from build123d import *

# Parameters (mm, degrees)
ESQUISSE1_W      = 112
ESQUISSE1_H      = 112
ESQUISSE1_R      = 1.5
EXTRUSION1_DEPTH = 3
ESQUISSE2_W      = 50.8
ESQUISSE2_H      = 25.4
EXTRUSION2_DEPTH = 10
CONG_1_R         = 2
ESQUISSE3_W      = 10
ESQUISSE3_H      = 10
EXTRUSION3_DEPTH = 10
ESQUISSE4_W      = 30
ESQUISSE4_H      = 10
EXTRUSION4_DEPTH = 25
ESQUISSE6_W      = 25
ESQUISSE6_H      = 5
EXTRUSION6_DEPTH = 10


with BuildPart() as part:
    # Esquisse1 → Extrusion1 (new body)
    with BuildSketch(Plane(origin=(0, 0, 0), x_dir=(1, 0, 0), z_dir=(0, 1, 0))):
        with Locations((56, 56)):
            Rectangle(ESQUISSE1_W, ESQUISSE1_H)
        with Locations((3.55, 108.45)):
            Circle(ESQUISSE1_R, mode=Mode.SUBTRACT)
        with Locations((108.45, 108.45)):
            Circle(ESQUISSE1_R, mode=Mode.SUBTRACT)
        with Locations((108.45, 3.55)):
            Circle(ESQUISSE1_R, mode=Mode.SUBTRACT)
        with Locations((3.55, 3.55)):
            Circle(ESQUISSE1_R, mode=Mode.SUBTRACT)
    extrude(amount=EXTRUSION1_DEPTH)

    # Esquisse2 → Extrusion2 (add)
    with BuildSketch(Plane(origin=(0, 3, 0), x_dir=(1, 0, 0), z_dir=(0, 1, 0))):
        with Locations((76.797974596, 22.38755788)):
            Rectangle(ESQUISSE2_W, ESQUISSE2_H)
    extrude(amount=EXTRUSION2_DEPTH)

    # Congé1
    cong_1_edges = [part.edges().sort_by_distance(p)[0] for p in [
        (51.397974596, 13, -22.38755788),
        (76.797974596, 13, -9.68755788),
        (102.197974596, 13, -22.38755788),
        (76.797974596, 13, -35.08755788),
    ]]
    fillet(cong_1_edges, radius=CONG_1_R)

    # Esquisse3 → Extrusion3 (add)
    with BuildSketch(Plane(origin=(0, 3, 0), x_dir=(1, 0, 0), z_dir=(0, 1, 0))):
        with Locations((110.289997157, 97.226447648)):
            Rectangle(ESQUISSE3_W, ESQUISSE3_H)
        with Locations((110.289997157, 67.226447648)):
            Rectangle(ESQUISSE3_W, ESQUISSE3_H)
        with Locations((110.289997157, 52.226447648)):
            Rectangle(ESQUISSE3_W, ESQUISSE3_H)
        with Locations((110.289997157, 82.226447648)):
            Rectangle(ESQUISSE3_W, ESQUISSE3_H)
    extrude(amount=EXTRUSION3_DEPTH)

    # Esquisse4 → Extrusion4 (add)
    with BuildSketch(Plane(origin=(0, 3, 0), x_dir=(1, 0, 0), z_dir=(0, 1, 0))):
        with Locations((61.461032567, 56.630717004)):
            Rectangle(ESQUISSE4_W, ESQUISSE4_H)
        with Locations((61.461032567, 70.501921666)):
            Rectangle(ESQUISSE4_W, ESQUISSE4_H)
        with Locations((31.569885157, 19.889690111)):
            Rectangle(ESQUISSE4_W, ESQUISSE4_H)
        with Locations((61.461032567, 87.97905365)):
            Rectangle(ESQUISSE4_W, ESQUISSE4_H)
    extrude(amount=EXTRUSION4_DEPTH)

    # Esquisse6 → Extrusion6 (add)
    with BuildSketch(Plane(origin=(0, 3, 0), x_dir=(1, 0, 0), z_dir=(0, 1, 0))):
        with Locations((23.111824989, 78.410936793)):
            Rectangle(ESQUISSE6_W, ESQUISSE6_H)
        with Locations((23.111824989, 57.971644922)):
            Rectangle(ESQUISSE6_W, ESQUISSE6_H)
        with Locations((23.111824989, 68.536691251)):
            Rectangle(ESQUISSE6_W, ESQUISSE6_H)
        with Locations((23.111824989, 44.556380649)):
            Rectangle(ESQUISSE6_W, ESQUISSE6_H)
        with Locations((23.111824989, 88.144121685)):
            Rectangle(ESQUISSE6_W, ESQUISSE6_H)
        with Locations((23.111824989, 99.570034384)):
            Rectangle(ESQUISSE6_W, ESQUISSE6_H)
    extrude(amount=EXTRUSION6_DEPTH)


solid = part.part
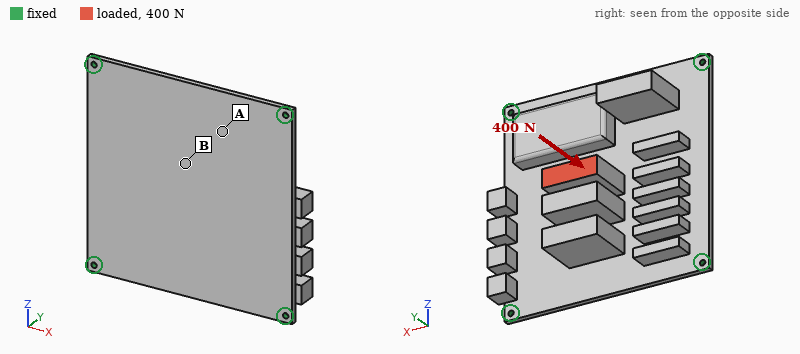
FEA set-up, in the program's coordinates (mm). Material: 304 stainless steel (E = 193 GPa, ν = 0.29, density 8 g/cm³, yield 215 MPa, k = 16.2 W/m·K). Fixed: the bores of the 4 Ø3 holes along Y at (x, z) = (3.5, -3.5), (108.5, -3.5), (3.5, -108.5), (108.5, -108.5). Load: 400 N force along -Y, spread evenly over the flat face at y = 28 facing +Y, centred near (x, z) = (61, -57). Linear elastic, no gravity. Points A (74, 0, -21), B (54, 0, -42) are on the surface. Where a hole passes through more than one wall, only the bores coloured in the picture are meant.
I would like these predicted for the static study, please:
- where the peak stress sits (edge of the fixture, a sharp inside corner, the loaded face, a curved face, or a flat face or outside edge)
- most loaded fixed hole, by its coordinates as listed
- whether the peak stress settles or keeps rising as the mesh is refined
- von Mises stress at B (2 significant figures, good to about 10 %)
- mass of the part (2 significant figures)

edge of the fixture
(108.5, -3.5)
keeps rising
30 MPa
730 g
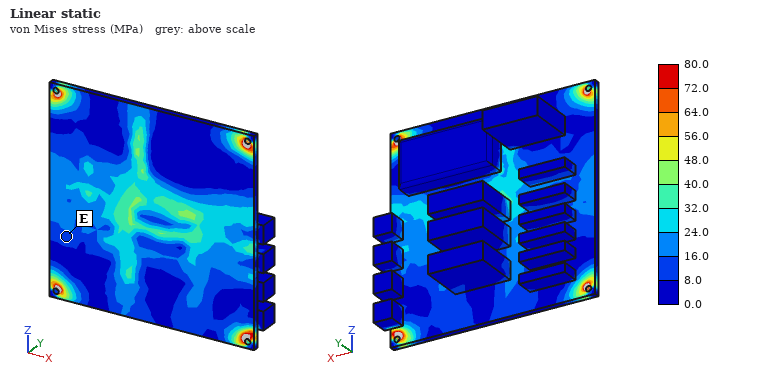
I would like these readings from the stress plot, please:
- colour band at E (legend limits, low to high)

8.0 to 16.0 MPa
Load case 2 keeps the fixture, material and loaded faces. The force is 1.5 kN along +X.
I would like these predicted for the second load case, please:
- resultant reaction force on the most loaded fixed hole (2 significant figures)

530 N
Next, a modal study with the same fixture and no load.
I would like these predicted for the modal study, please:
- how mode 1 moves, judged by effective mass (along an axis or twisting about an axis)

along Y
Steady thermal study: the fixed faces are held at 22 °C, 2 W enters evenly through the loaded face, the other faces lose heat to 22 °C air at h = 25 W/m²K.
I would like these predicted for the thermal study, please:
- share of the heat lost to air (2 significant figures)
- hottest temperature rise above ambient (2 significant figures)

92 %
15 K
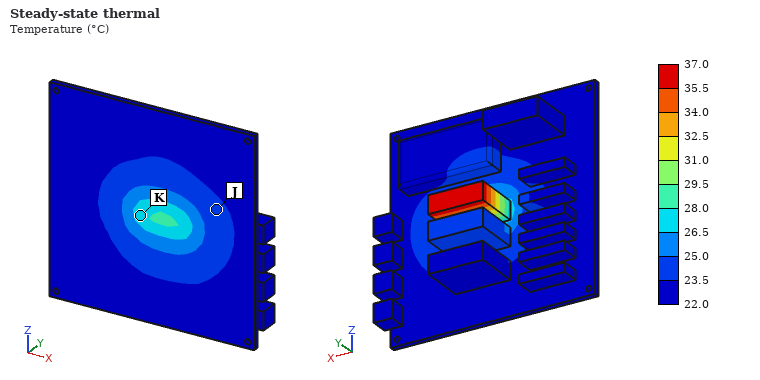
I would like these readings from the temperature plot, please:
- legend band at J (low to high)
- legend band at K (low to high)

23.5 to 25.0 °C
26.5 to 28.0 °C
